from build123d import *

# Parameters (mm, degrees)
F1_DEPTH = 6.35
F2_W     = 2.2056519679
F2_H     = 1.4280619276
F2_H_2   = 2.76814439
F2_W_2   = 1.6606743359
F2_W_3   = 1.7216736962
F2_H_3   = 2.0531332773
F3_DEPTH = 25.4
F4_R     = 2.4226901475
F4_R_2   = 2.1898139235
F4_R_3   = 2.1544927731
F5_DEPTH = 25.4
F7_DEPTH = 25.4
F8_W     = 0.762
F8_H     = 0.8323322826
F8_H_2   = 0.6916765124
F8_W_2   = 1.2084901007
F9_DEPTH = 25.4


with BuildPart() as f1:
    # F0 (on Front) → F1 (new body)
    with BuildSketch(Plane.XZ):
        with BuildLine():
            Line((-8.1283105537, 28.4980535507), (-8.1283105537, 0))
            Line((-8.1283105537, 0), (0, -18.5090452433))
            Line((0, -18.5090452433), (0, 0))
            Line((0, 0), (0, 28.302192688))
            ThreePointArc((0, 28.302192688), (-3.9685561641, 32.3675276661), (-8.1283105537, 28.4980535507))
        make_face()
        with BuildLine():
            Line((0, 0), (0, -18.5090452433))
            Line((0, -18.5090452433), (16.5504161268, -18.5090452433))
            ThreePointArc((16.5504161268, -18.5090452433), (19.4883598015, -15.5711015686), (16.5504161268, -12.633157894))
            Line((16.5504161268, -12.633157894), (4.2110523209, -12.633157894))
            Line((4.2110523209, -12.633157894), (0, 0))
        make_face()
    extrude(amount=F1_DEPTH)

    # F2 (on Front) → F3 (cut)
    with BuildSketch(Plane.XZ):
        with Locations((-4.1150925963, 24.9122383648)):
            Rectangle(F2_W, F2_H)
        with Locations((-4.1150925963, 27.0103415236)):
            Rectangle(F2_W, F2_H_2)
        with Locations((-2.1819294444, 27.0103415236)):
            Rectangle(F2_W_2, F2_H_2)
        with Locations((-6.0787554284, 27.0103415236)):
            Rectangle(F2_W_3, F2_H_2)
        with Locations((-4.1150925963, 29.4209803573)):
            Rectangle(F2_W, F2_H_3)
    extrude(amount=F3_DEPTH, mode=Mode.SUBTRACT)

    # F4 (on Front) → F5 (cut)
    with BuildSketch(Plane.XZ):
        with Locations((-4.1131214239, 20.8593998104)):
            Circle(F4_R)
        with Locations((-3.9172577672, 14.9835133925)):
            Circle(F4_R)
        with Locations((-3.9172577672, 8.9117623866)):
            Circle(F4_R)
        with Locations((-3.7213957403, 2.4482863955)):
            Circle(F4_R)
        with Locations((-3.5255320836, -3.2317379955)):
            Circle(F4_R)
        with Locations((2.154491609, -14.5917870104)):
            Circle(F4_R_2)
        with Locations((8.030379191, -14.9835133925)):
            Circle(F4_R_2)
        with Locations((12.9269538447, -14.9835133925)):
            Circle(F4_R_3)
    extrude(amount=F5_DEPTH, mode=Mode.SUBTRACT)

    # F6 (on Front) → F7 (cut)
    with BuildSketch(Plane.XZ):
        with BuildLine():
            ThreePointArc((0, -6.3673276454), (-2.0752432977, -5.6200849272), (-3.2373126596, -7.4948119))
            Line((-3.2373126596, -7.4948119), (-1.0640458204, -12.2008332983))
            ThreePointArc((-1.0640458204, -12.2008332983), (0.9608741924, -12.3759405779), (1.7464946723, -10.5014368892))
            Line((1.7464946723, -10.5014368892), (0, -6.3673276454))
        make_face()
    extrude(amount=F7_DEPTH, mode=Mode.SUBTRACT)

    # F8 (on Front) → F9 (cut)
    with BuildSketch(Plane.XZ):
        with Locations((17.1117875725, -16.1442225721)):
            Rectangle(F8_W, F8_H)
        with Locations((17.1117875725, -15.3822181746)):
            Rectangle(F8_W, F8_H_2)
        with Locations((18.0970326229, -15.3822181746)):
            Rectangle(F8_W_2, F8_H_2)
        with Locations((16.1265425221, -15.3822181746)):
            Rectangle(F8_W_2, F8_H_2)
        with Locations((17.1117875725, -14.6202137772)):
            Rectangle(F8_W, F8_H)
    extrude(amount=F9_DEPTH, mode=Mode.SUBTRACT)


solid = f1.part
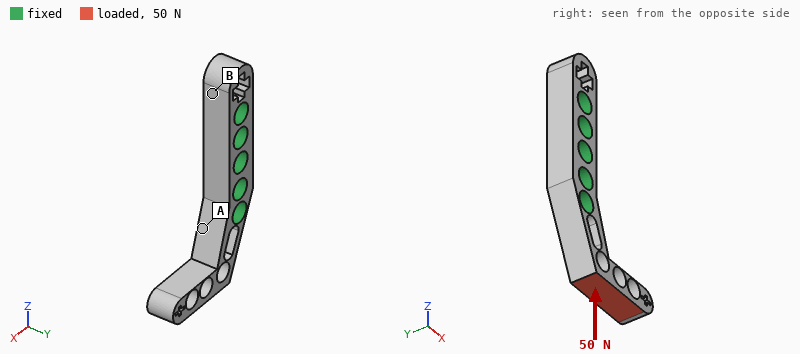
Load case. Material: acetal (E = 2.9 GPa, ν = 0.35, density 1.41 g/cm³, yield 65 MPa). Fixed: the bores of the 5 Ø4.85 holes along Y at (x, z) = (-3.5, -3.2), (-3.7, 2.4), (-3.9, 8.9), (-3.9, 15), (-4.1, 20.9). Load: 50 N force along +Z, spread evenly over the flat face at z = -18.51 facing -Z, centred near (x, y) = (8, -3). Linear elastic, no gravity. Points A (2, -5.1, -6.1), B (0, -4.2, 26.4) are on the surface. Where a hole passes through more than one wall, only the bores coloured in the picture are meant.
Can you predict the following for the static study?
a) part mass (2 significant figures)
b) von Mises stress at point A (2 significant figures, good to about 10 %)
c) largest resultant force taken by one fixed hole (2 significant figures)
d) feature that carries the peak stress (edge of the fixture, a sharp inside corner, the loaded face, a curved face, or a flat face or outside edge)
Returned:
2.5 g
18 MPa
31 N
a curved face
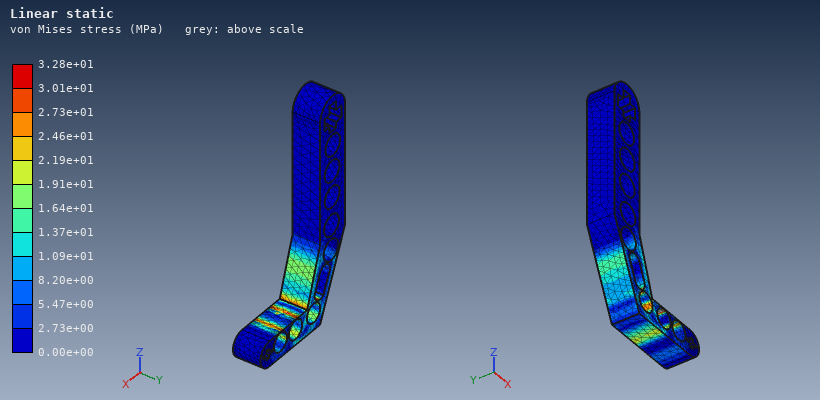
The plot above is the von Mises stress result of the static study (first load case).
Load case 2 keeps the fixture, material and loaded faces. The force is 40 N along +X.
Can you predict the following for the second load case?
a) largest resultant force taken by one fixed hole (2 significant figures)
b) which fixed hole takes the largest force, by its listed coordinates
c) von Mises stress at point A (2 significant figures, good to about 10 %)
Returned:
62 N
(-3.5, -3.2)
22 MPa
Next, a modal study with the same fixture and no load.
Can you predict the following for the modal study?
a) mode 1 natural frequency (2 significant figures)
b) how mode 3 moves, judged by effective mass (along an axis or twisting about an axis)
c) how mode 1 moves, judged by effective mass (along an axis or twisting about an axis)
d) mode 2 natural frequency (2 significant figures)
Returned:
1400 Hz
along X
along Y
1700 Hz
